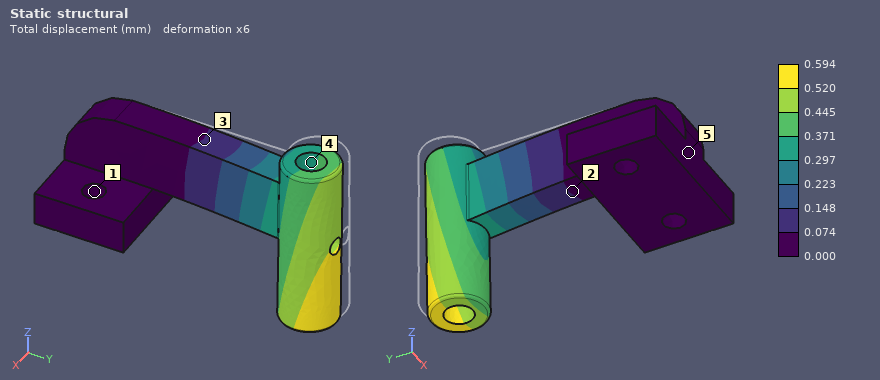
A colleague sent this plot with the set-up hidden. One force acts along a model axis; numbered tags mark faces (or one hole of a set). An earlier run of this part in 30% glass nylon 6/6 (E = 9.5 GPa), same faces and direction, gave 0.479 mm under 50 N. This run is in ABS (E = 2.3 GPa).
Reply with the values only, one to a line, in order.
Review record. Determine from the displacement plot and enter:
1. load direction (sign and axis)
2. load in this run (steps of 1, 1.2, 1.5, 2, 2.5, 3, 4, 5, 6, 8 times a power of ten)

+X
15 N
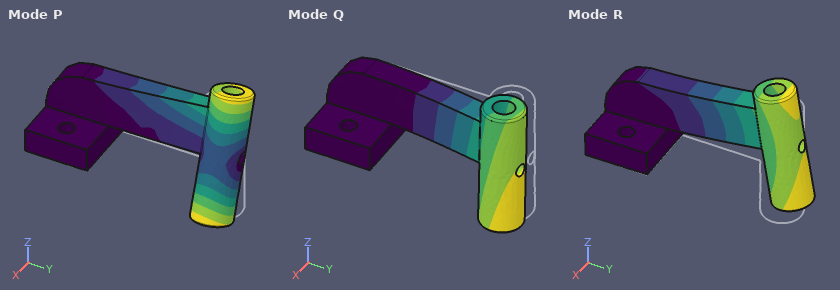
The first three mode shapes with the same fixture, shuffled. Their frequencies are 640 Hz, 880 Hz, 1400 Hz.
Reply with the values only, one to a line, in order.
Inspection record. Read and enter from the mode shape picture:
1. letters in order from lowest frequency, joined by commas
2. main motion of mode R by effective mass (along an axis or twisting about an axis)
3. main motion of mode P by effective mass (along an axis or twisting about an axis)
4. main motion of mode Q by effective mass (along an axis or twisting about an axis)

Q, R, P
along Z
twisting about Y
along X
